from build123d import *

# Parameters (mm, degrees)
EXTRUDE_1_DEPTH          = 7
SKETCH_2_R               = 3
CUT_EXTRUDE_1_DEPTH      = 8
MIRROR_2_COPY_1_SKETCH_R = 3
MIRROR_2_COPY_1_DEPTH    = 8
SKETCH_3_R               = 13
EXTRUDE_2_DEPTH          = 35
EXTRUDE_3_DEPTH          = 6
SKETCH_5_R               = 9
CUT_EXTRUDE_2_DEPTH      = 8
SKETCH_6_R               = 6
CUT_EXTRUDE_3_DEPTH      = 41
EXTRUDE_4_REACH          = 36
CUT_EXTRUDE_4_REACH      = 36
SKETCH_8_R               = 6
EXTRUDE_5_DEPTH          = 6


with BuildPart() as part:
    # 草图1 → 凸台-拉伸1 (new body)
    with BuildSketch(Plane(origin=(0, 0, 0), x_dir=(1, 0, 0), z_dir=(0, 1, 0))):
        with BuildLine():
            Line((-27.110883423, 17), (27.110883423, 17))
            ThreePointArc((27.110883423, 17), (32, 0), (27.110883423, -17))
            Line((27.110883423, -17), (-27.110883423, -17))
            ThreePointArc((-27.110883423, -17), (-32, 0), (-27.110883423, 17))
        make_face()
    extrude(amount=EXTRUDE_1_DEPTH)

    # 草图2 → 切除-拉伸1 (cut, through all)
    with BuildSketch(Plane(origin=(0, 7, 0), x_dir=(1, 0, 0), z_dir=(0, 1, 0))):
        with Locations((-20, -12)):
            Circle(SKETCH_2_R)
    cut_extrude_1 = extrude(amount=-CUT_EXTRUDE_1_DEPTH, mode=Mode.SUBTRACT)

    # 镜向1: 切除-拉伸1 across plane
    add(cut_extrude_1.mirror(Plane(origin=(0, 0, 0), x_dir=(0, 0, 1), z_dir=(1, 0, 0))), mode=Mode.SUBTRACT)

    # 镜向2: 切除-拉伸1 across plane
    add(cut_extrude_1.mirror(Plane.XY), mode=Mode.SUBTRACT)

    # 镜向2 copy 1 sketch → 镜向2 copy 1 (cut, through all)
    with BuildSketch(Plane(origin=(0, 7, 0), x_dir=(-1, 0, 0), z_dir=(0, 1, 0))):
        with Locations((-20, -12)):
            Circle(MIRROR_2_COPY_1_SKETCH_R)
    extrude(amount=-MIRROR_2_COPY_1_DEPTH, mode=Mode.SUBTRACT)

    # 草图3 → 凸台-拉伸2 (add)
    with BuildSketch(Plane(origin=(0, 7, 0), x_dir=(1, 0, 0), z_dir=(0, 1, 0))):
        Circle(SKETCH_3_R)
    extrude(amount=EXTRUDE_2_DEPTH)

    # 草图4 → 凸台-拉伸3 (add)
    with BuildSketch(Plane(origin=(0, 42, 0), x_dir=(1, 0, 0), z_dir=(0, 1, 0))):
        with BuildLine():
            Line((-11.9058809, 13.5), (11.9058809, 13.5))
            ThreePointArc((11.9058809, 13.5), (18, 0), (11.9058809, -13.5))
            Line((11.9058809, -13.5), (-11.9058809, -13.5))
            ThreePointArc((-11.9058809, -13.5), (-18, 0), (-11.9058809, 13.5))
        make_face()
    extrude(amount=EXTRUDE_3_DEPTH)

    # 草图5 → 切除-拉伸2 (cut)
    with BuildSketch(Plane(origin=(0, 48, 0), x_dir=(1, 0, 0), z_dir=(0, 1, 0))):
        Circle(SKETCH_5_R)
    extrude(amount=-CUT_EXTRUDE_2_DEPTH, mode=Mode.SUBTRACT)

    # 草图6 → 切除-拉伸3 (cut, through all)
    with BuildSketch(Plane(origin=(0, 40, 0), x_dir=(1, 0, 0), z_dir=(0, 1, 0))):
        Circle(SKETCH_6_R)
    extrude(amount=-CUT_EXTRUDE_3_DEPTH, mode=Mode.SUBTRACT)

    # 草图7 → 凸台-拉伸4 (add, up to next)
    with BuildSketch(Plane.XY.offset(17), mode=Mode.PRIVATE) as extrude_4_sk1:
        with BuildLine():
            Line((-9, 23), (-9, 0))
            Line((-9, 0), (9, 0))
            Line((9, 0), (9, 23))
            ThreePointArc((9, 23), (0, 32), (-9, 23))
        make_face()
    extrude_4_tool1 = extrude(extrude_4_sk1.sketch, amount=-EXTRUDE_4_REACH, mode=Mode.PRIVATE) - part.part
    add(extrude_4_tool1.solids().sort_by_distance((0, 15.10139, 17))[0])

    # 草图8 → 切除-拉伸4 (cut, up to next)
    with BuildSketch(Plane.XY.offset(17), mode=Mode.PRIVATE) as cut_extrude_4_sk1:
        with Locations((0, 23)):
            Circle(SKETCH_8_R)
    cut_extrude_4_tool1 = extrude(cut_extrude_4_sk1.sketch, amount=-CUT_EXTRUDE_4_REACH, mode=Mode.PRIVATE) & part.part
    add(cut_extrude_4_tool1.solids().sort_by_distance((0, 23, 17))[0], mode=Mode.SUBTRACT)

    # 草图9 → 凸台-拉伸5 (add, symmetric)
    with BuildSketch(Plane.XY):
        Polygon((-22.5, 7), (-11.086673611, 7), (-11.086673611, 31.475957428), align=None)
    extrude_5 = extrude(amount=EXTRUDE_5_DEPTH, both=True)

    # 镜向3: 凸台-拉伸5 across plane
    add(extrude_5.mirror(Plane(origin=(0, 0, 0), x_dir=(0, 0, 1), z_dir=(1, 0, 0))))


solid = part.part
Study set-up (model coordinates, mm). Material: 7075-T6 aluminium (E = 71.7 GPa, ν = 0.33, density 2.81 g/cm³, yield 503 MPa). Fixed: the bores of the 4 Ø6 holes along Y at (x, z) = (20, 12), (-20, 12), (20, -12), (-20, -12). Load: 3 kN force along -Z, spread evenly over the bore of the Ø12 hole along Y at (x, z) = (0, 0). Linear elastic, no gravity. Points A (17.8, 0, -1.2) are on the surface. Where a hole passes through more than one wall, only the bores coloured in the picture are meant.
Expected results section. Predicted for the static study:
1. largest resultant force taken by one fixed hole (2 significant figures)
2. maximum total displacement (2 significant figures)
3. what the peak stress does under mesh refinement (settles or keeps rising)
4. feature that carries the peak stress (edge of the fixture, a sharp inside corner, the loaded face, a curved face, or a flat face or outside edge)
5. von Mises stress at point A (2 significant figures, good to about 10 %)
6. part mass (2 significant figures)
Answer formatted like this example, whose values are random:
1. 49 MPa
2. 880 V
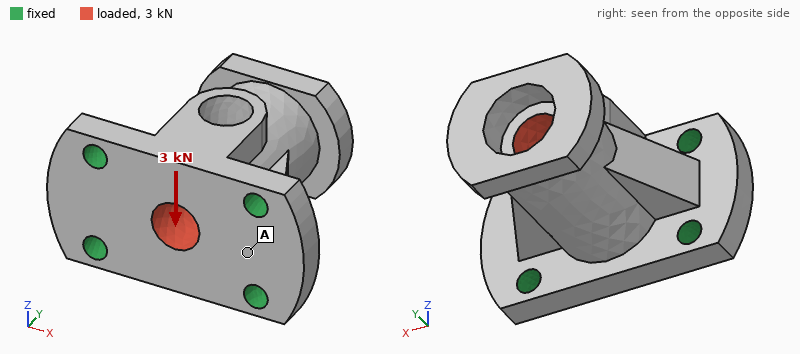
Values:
1. 1.4 kN
2. 41 µm
3. keeps rising
4. edge of the fixture
5. 6.8 MPa
6. 96 g
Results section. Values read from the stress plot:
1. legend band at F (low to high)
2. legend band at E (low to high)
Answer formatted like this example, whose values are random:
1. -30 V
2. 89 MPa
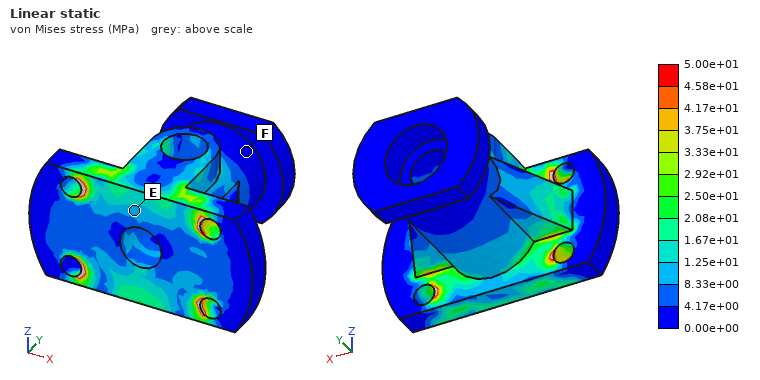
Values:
1. 0.00e+00 to 4.17e+00 MPa
2. 8.33e+00 to 1.25e+01 MPa
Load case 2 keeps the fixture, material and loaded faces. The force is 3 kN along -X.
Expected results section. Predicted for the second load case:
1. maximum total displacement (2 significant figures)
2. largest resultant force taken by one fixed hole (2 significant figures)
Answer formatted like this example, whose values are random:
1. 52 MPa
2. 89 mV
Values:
1. 13 µm
2. 1.0 kN
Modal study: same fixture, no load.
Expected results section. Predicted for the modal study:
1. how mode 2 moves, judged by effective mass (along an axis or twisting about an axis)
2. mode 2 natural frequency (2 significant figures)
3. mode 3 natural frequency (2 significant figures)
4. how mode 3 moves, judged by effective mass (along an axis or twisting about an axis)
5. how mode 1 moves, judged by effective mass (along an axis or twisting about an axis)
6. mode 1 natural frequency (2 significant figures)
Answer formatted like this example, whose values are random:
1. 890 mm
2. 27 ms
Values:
1. along X
2. 9100 Hz
3. 15 kHz
4. along Y
5. along Z
6. 5500 Hz
